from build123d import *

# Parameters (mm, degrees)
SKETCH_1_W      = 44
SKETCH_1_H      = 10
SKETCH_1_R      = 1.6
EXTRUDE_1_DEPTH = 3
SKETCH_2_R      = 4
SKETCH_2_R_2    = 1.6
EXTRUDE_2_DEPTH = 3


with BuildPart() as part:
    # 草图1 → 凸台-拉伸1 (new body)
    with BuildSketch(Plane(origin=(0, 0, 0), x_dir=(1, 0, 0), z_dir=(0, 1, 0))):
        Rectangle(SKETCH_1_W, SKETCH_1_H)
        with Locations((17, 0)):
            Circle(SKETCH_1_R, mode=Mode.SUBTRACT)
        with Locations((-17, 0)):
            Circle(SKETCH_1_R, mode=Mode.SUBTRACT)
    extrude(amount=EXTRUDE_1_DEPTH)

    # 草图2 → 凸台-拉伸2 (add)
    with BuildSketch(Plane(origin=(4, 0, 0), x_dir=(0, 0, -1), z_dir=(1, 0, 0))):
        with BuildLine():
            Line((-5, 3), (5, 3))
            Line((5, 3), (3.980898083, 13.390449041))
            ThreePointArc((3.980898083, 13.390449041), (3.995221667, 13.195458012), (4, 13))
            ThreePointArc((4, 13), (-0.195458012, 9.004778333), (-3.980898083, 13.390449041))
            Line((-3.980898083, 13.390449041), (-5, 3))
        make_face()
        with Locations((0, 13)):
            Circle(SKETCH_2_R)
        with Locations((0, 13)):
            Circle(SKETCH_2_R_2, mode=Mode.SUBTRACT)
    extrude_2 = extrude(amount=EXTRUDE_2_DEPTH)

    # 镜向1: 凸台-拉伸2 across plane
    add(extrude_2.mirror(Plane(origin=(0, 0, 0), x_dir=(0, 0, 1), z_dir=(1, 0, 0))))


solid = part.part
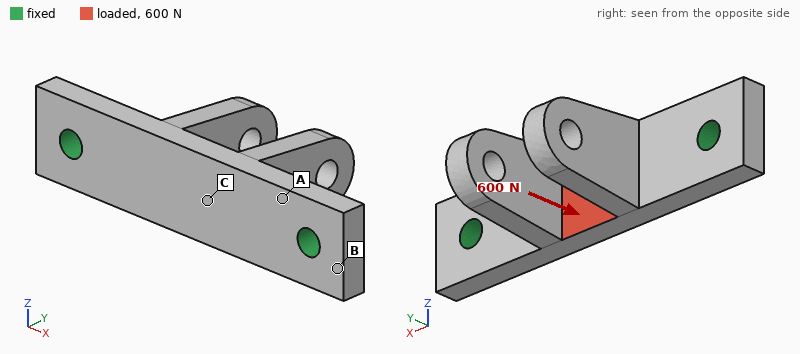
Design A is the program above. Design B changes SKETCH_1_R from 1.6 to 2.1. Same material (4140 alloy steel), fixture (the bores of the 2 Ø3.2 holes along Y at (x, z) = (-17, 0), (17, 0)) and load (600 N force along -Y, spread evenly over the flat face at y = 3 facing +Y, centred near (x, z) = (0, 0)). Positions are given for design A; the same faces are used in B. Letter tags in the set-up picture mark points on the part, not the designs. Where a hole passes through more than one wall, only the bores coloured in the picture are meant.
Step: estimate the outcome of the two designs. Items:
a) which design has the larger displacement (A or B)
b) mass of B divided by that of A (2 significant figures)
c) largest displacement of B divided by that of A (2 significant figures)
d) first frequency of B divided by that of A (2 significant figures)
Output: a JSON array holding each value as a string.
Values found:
["A", "0.98", "0.92", "1.0"]
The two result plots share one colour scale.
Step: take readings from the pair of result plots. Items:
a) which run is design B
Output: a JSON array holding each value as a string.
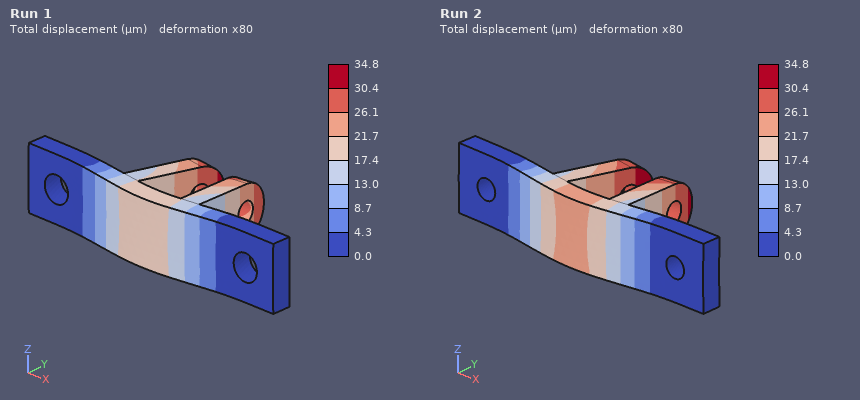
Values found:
["Run 1"]
